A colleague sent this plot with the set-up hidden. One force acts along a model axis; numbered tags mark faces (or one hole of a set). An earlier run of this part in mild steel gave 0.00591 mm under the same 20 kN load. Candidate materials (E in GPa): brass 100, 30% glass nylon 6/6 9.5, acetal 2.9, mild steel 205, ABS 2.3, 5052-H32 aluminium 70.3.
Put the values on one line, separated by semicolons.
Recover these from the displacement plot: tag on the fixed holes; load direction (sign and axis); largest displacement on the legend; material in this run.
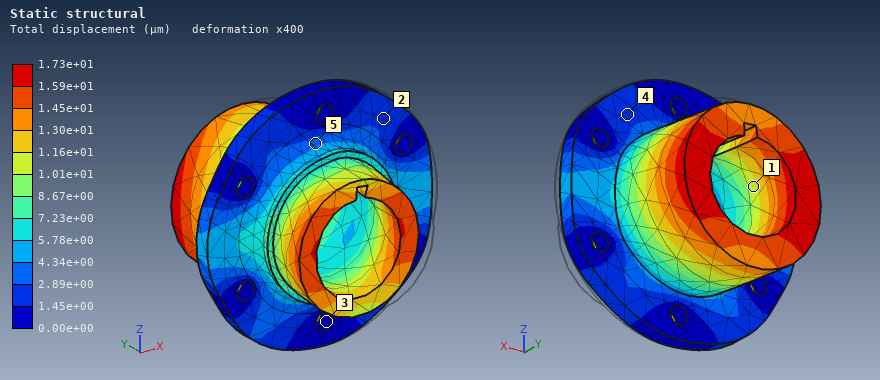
3; -X; 1.73e+01 µm; 5052-H32 aluminium
